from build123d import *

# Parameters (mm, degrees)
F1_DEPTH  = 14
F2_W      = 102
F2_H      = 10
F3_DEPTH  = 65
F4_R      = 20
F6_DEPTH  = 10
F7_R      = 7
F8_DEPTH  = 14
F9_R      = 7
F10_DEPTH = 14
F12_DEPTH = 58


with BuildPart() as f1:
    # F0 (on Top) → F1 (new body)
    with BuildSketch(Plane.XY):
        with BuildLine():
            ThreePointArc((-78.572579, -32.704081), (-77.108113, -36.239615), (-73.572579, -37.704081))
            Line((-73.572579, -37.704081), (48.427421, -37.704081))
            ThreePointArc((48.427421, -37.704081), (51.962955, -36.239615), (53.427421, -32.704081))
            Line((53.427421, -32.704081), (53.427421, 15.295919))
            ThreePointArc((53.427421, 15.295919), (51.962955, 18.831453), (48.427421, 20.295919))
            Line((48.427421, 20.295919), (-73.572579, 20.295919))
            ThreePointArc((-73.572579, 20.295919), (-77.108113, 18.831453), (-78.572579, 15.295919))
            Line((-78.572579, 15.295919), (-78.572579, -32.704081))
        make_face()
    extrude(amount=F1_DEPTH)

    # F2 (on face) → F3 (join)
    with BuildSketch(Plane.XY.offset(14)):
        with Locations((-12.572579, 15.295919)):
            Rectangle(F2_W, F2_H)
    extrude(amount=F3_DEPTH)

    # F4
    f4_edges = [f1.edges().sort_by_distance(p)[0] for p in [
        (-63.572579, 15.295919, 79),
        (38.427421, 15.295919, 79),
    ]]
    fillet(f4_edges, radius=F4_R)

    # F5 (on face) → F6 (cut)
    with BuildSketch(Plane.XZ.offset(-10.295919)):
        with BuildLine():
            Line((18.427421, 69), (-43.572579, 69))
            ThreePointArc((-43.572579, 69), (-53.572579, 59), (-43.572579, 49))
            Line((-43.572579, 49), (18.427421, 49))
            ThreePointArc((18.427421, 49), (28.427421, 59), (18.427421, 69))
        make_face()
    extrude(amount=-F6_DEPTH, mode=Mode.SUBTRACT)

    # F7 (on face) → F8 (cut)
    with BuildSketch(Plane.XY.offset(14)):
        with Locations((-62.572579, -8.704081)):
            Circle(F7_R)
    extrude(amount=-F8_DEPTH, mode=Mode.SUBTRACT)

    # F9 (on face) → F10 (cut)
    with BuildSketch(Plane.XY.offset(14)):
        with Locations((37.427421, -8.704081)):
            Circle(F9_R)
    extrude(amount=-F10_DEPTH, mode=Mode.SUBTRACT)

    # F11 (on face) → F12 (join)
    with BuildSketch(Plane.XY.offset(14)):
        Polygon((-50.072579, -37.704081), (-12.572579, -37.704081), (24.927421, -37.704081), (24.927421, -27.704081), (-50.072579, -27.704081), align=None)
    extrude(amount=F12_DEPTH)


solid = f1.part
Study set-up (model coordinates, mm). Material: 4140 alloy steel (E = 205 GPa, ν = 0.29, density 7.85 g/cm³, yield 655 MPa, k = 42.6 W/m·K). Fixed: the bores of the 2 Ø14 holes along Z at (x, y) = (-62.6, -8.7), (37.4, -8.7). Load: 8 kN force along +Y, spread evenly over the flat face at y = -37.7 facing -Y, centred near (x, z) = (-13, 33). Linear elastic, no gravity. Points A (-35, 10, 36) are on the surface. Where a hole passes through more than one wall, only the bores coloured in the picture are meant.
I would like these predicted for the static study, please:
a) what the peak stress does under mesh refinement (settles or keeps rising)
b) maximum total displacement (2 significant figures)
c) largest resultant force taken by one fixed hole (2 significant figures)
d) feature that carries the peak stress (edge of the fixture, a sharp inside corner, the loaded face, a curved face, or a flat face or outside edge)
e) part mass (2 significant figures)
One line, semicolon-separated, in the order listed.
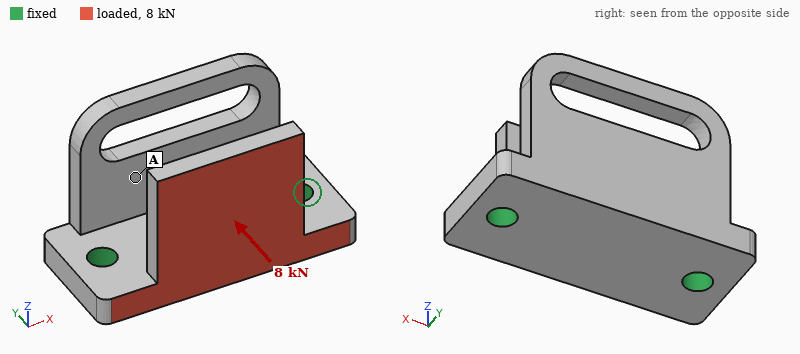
keeps rising; 0.22 mm; 4.0 kN; a sharp inside corner; 1.5 kg
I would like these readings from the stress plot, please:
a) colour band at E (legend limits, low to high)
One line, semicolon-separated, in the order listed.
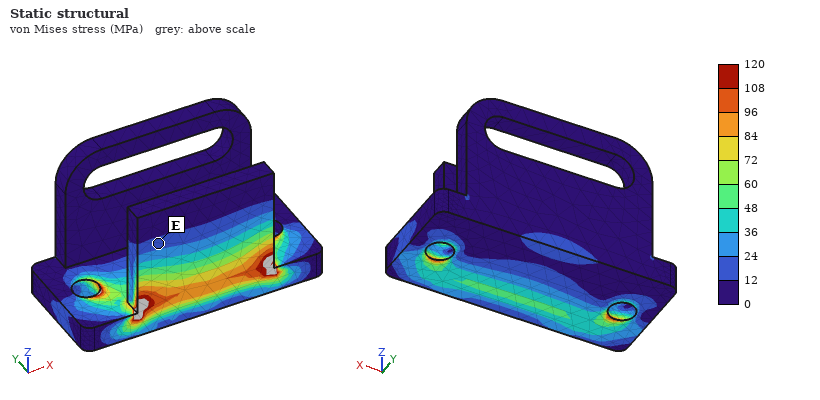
12 to 24 MPa
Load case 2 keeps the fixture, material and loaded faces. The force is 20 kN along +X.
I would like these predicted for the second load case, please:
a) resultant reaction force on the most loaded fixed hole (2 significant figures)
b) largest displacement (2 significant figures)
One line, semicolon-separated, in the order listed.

13 kN; 52 µm
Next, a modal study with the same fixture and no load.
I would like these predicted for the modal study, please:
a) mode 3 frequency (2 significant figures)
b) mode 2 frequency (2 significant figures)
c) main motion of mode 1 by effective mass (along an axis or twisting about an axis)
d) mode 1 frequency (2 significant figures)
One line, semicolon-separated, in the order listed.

3000 Hz; 1800 Hz; along Y; 1600 Hz
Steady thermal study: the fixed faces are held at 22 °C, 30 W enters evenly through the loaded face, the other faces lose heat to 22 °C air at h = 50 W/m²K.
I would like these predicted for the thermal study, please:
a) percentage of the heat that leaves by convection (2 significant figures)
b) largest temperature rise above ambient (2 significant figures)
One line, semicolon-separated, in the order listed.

37 %; 26 K
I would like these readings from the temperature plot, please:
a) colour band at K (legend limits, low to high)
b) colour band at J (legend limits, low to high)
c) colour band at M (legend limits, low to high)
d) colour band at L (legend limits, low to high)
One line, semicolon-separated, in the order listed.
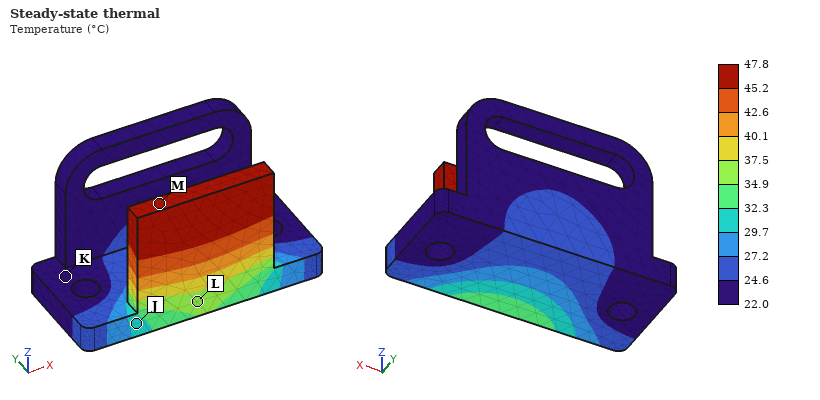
22.0 to 24.6 °C; 29.7 to 32.3 °C; 45.2 to 47.8 °C; 34.9 to 37.5 °C
